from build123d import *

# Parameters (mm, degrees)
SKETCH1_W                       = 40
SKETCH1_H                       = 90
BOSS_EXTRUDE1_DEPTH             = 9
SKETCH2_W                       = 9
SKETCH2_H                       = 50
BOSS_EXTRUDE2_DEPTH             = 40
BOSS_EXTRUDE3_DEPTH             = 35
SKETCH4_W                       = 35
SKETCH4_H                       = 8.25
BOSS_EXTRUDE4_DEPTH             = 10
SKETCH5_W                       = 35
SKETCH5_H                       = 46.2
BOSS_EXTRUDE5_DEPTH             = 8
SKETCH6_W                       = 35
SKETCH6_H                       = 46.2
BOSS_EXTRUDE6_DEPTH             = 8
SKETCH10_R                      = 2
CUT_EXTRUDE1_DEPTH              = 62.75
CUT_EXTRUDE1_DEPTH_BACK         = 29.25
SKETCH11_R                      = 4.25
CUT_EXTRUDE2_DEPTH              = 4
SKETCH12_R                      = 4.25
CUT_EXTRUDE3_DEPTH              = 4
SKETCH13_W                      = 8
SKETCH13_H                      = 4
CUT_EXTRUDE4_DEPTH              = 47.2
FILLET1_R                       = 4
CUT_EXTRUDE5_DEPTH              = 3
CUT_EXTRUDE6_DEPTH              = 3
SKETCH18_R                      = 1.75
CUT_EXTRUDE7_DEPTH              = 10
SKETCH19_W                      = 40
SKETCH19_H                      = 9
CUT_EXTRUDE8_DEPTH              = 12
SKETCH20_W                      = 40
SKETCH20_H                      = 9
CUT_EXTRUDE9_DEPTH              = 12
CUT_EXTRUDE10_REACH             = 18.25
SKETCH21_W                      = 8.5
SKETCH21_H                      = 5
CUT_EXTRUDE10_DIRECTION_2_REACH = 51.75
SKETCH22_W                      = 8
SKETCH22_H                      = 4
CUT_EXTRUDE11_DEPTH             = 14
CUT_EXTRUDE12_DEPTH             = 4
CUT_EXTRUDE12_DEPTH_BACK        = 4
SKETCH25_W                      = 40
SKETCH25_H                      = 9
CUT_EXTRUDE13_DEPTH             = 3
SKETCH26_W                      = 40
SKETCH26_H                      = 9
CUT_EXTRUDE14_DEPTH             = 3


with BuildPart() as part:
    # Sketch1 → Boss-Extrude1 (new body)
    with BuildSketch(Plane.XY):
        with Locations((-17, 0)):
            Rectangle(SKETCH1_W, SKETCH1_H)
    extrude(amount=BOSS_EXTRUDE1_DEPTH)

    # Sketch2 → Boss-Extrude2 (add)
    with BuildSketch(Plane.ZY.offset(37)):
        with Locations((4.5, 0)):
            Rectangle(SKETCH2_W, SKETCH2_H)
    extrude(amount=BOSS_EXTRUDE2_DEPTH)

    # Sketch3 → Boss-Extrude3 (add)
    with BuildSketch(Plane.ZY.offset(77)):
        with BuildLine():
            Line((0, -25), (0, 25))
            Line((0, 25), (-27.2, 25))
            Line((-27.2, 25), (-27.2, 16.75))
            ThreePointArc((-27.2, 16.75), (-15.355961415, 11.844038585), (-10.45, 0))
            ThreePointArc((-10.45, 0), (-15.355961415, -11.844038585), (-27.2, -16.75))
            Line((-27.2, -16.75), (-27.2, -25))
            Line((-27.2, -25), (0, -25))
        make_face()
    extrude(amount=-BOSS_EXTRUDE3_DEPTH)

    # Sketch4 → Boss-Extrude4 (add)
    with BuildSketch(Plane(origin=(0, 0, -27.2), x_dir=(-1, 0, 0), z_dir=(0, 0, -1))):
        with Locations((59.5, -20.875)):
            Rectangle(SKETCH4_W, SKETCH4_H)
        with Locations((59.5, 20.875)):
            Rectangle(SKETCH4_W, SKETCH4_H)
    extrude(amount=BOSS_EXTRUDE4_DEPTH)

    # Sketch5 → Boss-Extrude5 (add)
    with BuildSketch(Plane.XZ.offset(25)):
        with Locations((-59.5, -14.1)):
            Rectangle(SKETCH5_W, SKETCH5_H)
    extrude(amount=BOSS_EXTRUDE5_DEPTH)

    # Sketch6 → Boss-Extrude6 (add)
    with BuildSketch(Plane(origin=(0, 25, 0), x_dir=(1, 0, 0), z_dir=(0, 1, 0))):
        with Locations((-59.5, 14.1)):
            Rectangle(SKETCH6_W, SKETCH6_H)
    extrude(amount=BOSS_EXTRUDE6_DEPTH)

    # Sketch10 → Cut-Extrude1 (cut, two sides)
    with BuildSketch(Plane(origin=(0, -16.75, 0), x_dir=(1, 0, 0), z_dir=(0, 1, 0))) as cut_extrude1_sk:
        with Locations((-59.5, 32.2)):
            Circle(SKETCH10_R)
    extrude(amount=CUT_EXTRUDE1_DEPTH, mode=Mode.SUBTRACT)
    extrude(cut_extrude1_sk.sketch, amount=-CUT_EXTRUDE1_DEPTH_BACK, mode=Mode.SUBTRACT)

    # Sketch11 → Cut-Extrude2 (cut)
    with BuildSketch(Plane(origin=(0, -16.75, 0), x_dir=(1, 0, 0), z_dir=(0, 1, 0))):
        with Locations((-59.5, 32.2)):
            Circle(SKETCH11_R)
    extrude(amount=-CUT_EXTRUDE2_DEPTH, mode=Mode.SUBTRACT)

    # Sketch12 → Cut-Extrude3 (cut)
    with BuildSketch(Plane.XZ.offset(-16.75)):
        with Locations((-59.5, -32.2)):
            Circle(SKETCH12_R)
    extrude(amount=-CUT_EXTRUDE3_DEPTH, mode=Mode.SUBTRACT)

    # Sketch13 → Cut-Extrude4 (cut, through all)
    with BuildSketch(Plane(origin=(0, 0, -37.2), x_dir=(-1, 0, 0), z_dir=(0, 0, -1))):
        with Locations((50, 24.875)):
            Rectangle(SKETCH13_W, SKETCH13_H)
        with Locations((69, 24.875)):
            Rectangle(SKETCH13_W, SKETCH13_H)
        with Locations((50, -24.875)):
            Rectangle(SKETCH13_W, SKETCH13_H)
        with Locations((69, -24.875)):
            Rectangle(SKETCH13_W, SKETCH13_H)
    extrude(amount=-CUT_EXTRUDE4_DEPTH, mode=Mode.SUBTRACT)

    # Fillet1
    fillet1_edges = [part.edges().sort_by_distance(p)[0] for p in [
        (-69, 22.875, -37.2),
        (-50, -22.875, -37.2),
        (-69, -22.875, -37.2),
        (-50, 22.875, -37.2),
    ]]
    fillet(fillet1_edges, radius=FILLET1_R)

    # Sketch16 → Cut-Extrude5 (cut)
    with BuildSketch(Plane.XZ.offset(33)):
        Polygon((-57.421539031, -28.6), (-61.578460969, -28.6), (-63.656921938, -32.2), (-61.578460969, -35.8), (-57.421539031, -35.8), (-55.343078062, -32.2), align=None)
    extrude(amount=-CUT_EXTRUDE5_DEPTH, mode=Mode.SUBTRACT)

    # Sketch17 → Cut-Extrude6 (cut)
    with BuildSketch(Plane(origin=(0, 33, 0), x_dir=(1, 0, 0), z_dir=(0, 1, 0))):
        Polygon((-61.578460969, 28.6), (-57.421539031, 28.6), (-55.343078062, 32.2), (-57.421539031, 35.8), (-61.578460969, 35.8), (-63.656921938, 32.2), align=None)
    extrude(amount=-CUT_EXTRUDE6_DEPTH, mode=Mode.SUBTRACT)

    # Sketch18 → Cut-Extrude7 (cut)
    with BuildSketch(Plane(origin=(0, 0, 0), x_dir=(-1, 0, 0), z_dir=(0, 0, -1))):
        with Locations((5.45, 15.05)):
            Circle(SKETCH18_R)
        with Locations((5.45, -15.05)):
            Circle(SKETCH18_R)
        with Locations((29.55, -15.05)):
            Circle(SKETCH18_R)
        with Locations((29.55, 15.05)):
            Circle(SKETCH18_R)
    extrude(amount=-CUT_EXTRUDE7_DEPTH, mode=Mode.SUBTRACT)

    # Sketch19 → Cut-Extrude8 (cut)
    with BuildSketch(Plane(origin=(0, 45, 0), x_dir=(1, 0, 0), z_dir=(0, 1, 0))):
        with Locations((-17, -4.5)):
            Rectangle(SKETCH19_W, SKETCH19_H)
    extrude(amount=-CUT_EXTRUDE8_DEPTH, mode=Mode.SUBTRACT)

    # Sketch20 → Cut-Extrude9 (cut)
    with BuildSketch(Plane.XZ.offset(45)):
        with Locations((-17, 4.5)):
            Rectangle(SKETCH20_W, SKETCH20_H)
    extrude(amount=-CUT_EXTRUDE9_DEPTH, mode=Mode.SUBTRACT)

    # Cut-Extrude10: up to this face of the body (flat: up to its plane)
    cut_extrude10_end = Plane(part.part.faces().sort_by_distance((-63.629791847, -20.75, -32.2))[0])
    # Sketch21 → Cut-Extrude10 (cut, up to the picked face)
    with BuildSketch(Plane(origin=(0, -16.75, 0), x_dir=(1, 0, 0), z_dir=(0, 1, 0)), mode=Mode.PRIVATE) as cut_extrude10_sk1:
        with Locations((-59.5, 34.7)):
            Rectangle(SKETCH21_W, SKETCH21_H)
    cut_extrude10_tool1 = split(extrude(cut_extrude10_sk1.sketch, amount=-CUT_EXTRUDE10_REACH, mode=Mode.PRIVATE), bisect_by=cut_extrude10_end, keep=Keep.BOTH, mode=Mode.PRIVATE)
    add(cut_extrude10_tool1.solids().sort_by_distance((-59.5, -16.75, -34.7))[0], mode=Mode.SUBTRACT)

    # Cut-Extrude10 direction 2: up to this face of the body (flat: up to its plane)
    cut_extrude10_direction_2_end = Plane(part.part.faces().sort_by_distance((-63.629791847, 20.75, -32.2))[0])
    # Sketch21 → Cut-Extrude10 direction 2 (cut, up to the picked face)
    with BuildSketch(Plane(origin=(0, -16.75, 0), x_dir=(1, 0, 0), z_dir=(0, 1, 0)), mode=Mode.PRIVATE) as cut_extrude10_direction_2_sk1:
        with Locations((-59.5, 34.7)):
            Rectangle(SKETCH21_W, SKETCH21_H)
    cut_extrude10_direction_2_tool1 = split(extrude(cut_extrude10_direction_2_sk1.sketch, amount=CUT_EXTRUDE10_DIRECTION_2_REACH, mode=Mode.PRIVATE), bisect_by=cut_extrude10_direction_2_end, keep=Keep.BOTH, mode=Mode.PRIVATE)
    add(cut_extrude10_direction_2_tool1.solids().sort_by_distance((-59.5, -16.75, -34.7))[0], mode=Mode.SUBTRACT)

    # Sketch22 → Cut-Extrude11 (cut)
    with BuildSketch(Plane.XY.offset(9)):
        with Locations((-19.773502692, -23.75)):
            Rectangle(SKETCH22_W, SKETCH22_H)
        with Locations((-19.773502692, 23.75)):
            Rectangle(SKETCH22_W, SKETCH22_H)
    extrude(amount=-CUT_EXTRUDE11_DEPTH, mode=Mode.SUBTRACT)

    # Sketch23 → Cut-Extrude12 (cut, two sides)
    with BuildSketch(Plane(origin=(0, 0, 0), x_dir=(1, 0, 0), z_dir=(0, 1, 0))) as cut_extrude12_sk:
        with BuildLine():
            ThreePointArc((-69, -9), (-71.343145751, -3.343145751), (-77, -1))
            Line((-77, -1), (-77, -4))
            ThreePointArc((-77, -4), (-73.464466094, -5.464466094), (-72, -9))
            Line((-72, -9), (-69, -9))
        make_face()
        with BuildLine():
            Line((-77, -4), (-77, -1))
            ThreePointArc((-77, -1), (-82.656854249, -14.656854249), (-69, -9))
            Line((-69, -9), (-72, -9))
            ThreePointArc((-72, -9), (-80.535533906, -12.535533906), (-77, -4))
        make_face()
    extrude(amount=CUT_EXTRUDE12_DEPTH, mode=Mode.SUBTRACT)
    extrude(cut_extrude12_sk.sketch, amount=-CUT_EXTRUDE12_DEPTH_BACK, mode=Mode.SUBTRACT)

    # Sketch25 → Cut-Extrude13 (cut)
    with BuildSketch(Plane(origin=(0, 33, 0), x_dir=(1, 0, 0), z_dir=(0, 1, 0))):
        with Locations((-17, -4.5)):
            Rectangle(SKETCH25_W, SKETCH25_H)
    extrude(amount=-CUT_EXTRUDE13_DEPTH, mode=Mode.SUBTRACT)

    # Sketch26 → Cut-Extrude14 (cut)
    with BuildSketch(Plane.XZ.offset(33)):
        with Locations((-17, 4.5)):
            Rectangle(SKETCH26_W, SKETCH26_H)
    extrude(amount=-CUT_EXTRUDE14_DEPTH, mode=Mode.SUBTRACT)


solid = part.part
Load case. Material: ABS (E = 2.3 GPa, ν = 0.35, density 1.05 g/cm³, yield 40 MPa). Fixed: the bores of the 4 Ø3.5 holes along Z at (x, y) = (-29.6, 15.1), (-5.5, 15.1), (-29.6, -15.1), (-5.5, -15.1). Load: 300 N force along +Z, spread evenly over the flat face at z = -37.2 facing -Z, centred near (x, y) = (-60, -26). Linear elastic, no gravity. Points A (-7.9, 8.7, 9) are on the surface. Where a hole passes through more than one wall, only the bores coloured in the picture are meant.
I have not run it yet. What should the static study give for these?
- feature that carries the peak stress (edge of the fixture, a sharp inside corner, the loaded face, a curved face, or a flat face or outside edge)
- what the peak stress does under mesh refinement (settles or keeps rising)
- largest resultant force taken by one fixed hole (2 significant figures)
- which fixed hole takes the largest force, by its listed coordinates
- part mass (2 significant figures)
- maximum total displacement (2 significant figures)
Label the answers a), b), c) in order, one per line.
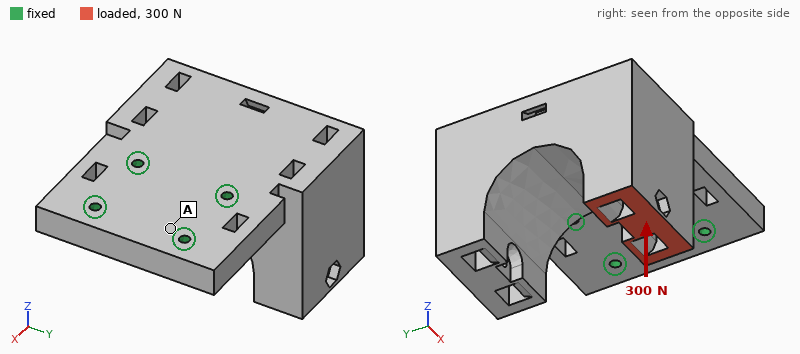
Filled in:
a) edge of the fixture
b) keeps rising
c) 460 N
d) (-29.6, -15.1)
e) 100 g
f) 1.2 mm
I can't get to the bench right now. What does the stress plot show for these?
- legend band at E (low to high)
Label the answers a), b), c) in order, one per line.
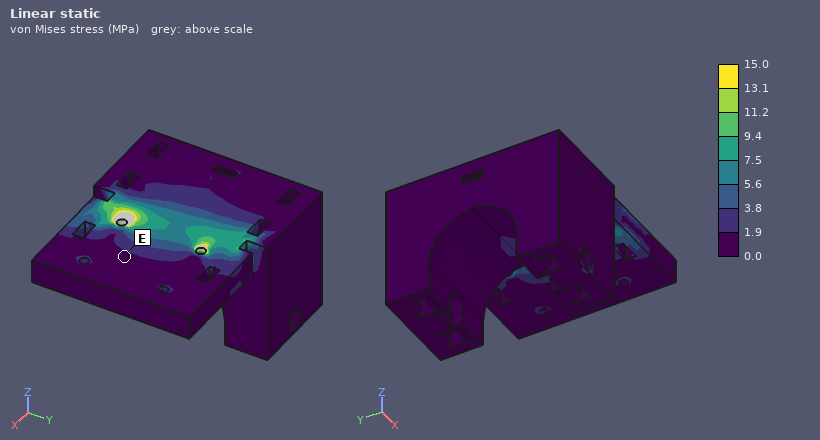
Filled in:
a) 0.0 to 1.9 MPa
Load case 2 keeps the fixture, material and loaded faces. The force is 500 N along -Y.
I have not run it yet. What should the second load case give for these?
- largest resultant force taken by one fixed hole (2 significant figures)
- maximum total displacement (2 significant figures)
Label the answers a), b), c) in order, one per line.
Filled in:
a) 770 N
b) 0.95 mm
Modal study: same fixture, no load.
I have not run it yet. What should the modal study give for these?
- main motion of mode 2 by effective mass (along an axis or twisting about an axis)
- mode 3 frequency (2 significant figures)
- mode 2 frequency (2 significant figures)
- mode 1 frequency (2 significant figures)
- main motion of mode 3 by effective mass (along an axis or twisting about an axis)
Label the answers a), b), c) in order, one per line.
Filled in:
a) along Y
b) 1400 Hz
c) 820 Hz
d) 370 Hz
e) along Y
